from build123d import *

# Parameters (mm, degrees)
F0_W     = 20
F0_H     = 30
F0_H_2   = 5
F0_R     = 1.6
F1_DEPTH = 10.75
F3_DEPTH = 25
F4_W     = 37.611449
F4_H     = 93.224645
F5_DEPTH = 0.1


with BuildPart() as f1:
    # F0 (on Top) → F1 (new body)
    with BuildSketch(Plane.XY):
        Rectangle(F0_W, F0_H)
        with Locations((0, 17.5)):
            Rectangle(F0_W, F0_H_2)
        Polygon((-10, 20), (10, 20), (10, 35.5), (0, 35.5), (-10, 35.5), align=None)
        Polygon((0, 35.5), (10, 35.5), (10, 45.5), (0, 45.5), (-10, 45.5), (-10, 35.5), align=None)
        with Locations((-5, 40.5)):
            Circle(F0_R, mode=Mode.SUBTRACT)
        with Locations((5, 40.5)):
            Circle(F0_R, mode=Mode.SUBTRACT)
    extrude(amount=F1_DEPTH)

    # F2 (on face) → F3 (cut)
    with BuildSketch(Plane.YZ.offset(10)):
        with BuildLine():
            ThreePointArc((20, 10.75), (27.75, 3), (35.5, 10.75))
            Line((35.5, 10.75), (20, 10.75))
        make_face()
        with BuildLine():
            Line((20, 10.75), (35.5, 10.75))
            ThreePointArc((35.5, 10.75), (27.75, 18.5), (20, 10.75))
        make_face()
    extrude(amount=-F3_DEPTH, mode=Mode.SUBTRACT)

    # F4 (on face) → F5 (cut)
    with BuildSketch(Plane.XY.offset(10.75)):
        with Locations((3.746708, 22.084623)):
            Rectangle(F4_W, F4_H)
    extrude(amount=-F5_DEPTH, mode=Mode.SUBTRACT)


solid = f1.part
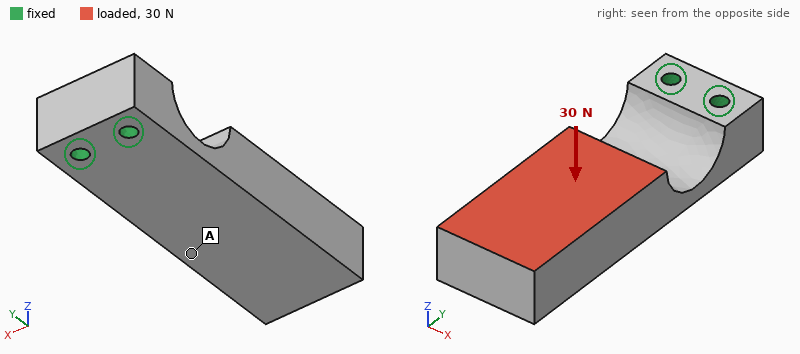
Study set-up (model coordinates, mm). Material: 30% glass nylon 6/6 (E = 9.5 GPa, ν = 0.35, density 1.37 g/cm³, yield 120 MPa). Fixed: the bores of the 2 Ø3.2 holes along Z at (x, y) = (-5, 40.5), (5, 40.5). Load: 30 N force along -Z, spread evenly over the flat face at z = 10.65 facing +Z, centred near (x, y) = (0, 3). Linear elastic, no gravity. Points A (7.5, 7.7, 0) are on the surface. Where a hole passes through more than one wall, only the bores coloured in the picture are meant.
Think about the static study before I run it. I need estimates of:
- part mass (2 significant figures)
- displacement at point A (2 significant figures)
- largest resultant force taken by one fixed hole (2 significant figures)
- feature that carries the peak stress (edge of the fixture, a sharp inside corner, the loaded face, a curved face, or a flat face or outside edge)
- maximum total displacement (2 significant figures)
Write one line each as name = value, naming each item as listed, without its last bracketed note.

part mass = 15 g
displacement at point A = 0.30 mm
largest resultant force taken by one fixed hole = 15 N
feature that carries the peak stress = a flat face or outside edge
maximum total displacement = 0.64 mm
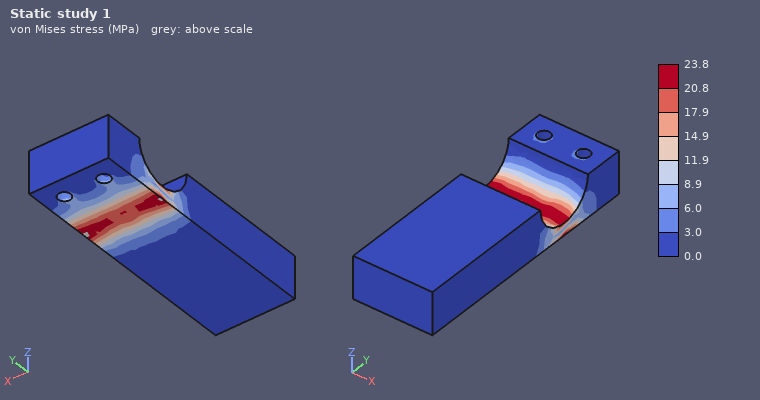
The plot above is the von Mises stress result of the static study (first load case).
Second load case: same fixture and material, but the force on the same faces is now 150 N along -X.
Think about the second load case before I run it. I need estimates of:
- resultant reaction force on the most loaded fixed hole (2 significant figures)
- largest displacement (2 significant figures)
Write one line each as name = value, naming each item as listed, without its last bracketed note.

resultant reaction force on the most loaded fixed hole = 470 N
largest displacement = 0.30 mm
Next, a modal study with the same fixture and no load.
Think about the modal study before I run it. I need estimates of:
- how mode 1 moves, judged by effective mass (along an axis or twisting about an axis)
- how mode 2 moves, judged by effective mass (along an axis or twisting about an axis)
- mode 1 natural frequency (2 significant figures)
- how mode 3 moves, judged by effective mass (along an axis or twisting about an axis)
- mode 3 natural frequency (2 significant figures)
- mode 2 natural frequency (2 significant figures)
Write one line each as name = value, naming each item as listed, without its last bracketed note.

how mode 1 moves, judged by effective mass = along Z
how mode 2 moves, judged by effective mass = along X
mode 1 natural frequency = 410 Hz
how mode 3 moves, judged by effective mass = twisting about Y
mode 3 natural frequency = 2900 Hz
mode 2 natural frequency = 1500 Hz
